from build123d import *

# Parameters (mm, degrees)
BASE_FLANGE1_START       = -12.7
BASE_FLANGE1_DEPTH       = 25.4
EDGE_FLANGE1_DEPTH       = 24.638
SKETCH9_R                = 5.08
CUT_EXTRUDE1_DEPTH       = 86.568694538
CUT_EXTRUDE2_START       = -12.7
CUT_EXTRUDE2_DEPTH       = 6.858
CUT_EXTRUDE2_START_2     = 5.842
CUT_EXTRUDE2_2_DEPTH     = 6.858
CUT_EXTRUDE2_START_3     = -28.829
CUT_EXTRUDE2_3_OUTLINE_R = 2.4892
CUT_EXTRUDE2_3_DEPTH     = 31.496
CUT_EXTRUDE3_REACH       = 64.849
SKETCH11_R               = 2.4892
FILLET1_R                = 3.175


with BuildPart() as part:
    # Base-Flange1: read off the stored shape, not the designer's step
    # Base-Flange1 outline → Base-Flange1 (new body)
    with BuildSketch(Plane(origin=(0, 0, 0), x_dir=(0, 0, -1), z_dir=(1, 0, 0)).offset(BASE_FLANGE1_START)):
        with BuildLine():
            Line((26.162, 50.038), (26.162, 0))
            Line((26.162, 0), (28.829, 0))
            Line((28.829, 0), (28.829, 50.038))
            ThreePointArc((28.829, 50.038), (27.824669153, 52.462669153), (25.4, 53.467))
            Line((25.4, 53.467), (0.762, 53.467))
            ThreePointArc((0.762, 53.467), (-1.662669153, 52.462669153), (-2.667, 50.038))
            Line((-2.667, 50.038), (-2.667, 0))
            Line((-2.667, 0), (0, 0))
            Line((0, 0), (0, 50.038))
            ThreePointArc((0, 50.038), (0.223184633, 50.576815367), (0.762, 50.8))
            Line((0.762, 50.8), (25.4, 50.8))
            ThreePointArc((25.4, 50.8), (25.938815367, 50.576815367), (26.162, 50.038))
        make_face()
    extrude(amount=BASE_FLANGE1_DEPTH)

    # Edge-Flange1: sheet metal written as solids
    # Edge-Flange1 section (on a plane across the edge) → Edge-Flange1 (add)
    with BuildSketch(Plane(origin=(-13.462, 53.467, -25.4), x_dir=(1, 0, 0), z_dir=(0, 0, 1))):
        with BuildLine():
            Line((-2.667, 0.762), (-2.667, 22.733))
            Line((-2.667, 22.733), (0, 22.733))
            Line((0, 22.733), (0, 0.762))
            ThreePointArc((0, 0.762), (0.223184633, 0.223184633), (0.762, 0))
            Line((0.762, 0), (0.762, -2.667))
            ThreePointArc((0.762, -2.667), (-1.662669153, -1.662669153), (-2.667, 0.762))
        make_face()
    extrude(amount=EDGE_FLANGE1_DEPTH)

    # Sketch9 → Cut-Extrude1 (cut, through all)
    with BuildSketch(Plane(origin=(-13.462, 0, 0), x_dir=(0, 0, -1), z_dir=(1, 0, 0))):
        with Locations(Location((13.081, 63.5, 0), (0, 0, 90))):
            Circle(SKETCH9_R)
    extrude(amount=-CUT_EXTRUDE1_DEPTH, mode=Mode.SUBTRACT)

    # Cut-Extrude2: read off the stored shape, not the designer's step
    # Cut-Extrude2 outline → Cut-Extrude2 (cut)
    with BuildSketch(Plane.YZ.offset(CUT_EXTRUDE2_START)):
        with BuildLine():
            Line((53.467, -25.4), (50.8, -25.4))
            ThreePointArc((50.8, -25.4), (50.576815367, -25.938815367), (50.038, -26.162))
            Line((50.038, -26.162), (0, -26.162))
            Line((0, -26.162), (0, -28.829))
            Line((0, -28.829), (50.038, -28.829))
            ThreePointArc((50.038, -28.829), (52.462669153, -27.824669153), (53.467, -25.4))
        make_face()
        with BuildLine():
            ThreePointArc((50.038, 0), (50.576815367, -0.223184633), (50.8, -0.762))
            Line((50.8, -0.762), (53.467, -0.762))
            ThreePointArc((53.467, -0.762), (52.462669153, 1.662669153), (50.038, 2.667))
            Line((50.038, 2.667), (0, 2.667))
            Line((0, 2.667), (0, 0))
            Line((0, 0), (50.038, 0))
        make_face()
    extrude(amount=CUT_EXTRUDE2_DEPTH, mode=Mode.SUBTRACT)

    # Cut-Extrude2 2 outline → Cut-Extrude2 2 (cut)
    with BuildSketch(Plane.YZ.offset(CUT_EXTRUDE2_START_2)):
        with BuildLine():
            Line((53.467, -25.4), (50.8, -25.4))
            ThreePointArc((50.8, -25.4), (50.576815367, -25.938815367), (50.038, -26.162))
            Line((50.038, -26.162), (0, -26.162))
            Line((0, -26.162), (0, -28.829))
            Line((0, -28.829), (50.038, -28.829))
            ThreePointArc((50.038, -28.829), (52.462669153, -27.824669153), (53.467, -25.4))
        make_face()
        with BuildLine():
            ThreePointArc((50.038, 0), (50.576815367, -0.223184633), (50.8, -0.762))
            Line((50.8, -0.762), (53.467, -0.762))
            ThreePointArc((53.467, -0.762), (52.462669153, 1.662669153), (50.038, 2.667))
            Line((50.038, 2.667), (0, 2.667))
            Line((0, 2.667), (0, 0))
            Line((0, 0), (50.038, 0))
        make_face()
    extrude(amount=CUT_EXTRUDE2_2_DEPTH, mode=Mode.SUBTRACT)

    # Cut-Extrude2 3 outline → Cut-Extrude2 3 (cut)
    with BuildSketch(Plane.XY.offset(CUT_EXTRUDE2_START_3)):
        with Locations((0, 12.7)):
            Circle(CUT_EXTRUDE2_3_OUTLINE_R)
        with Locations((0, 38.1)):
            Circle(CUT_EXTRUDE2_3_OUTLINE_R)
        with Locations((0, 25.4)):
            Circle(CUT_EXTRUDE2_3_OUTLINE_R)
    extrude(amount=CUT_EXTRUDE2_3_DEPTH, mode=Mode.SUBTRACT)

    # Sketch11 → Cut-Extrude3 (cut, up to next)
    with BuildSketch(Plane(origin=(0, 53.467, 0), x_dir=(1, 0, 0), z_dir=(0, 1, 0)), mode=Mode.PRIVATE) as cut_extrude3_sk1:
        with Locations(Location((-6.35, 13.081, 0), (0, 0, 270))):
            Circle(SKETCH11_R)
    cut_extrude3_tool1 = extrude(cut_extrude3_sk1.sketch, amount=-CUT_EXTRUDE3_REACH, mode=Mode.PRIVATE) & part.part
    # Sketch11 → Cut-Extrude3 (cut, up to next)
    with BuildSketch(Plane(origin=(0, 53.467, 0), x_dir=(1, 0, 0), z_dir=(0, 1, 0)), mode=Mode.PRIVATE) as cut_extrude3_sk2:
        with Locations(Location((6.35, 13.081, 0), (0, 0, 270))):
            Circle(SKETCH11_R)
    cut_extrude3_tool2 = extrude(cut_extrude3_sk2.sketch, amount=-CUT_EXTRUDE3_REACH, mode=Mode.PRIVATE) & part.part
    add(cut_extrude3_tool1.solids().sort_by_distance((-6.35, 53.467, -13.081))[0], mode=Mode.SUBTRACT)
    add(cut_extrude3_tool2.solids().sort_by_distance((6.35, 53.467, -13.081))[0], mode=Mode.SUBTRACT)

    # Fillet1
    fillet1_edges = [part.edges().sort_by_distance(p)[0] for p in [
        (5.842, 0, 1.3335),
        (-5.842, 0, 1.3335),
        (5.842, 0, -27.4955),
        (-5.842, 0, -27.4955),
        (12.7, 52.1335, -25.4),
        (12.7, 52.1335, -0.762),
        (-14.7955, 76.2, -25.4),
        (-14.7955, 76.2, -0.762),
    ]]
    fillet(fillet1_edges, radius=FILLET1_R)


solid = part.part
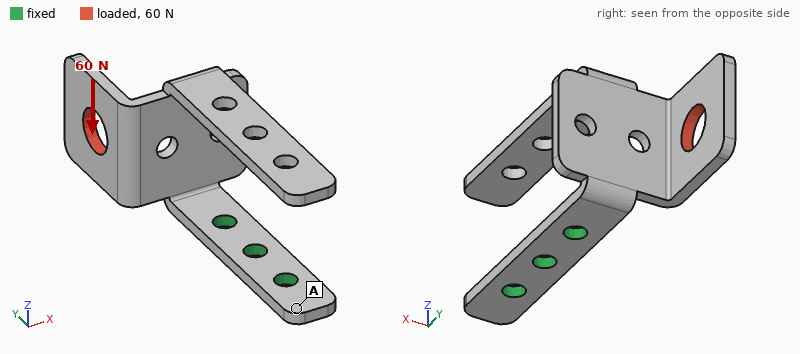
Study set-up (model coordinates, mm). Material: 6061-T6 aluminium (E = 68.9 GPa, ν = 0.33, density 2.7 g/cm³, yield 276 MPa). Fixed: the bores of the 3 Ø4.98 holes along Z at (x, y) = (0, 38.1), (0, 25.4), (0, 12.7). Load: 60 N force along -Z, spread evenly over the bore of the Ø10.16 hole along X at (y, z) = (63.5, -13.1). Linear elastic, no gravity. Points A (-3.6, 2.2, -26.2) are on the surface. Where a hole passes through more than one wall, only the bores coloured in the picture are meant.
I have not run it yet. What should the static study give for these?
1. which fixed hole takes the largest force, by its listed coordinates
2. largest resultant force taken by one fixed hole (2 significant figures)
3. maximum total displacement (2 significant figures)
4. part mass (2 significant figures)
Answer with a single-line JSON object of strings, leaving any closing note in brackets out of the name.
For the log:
{"which fixed hole takes the largest force, by its listed coordinates": "(0, 38.1)", "largest resultant force taken by one fixed hole": "62 N", "maximum total displacement": "0.85 mm", "part mass": "16 g"}
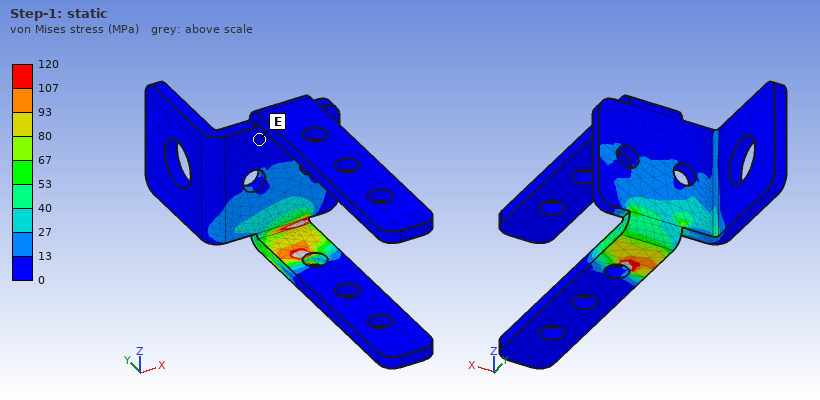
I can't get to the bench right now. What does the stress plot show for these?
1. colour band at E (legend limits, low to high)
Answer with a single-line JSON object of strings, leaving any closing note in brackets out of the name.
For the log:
{"colour band at E": "0 to 13 MPa"}
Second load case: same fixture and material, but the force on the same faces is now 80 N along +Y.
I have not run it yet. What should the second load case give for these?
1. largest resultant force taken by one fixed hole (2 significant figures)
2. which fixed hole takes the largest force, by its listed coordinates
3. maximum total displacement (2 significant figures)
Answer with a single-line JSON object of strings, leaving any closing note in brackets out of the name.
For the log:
{"largest resultant force taken by one fixed hole": "79 N", "which fixed hole takes the largest force, by its listed coordinates": "(0, 38.1)", "maximum total displacement": "0.93 mm"}
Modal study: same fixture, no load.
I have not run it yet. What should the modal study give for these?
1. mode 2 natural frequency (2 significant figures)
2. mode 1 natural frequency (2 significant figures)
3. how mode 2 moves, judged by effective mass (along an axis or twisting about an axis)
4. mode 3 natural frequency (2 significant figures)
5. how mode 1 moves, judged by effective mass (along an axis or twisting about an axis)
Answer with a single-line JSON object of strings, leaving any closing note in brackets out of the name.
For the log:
{"mode 2 natural frequency": "590 Hz", "mode 1 natural frequency": "390 Hz", "how mode 2 moves, judged by effective mass": "along X", "mode 3 natural frequency": "880 Hz", "how mode 1 moves, judged by effective mass": "along Y"}
